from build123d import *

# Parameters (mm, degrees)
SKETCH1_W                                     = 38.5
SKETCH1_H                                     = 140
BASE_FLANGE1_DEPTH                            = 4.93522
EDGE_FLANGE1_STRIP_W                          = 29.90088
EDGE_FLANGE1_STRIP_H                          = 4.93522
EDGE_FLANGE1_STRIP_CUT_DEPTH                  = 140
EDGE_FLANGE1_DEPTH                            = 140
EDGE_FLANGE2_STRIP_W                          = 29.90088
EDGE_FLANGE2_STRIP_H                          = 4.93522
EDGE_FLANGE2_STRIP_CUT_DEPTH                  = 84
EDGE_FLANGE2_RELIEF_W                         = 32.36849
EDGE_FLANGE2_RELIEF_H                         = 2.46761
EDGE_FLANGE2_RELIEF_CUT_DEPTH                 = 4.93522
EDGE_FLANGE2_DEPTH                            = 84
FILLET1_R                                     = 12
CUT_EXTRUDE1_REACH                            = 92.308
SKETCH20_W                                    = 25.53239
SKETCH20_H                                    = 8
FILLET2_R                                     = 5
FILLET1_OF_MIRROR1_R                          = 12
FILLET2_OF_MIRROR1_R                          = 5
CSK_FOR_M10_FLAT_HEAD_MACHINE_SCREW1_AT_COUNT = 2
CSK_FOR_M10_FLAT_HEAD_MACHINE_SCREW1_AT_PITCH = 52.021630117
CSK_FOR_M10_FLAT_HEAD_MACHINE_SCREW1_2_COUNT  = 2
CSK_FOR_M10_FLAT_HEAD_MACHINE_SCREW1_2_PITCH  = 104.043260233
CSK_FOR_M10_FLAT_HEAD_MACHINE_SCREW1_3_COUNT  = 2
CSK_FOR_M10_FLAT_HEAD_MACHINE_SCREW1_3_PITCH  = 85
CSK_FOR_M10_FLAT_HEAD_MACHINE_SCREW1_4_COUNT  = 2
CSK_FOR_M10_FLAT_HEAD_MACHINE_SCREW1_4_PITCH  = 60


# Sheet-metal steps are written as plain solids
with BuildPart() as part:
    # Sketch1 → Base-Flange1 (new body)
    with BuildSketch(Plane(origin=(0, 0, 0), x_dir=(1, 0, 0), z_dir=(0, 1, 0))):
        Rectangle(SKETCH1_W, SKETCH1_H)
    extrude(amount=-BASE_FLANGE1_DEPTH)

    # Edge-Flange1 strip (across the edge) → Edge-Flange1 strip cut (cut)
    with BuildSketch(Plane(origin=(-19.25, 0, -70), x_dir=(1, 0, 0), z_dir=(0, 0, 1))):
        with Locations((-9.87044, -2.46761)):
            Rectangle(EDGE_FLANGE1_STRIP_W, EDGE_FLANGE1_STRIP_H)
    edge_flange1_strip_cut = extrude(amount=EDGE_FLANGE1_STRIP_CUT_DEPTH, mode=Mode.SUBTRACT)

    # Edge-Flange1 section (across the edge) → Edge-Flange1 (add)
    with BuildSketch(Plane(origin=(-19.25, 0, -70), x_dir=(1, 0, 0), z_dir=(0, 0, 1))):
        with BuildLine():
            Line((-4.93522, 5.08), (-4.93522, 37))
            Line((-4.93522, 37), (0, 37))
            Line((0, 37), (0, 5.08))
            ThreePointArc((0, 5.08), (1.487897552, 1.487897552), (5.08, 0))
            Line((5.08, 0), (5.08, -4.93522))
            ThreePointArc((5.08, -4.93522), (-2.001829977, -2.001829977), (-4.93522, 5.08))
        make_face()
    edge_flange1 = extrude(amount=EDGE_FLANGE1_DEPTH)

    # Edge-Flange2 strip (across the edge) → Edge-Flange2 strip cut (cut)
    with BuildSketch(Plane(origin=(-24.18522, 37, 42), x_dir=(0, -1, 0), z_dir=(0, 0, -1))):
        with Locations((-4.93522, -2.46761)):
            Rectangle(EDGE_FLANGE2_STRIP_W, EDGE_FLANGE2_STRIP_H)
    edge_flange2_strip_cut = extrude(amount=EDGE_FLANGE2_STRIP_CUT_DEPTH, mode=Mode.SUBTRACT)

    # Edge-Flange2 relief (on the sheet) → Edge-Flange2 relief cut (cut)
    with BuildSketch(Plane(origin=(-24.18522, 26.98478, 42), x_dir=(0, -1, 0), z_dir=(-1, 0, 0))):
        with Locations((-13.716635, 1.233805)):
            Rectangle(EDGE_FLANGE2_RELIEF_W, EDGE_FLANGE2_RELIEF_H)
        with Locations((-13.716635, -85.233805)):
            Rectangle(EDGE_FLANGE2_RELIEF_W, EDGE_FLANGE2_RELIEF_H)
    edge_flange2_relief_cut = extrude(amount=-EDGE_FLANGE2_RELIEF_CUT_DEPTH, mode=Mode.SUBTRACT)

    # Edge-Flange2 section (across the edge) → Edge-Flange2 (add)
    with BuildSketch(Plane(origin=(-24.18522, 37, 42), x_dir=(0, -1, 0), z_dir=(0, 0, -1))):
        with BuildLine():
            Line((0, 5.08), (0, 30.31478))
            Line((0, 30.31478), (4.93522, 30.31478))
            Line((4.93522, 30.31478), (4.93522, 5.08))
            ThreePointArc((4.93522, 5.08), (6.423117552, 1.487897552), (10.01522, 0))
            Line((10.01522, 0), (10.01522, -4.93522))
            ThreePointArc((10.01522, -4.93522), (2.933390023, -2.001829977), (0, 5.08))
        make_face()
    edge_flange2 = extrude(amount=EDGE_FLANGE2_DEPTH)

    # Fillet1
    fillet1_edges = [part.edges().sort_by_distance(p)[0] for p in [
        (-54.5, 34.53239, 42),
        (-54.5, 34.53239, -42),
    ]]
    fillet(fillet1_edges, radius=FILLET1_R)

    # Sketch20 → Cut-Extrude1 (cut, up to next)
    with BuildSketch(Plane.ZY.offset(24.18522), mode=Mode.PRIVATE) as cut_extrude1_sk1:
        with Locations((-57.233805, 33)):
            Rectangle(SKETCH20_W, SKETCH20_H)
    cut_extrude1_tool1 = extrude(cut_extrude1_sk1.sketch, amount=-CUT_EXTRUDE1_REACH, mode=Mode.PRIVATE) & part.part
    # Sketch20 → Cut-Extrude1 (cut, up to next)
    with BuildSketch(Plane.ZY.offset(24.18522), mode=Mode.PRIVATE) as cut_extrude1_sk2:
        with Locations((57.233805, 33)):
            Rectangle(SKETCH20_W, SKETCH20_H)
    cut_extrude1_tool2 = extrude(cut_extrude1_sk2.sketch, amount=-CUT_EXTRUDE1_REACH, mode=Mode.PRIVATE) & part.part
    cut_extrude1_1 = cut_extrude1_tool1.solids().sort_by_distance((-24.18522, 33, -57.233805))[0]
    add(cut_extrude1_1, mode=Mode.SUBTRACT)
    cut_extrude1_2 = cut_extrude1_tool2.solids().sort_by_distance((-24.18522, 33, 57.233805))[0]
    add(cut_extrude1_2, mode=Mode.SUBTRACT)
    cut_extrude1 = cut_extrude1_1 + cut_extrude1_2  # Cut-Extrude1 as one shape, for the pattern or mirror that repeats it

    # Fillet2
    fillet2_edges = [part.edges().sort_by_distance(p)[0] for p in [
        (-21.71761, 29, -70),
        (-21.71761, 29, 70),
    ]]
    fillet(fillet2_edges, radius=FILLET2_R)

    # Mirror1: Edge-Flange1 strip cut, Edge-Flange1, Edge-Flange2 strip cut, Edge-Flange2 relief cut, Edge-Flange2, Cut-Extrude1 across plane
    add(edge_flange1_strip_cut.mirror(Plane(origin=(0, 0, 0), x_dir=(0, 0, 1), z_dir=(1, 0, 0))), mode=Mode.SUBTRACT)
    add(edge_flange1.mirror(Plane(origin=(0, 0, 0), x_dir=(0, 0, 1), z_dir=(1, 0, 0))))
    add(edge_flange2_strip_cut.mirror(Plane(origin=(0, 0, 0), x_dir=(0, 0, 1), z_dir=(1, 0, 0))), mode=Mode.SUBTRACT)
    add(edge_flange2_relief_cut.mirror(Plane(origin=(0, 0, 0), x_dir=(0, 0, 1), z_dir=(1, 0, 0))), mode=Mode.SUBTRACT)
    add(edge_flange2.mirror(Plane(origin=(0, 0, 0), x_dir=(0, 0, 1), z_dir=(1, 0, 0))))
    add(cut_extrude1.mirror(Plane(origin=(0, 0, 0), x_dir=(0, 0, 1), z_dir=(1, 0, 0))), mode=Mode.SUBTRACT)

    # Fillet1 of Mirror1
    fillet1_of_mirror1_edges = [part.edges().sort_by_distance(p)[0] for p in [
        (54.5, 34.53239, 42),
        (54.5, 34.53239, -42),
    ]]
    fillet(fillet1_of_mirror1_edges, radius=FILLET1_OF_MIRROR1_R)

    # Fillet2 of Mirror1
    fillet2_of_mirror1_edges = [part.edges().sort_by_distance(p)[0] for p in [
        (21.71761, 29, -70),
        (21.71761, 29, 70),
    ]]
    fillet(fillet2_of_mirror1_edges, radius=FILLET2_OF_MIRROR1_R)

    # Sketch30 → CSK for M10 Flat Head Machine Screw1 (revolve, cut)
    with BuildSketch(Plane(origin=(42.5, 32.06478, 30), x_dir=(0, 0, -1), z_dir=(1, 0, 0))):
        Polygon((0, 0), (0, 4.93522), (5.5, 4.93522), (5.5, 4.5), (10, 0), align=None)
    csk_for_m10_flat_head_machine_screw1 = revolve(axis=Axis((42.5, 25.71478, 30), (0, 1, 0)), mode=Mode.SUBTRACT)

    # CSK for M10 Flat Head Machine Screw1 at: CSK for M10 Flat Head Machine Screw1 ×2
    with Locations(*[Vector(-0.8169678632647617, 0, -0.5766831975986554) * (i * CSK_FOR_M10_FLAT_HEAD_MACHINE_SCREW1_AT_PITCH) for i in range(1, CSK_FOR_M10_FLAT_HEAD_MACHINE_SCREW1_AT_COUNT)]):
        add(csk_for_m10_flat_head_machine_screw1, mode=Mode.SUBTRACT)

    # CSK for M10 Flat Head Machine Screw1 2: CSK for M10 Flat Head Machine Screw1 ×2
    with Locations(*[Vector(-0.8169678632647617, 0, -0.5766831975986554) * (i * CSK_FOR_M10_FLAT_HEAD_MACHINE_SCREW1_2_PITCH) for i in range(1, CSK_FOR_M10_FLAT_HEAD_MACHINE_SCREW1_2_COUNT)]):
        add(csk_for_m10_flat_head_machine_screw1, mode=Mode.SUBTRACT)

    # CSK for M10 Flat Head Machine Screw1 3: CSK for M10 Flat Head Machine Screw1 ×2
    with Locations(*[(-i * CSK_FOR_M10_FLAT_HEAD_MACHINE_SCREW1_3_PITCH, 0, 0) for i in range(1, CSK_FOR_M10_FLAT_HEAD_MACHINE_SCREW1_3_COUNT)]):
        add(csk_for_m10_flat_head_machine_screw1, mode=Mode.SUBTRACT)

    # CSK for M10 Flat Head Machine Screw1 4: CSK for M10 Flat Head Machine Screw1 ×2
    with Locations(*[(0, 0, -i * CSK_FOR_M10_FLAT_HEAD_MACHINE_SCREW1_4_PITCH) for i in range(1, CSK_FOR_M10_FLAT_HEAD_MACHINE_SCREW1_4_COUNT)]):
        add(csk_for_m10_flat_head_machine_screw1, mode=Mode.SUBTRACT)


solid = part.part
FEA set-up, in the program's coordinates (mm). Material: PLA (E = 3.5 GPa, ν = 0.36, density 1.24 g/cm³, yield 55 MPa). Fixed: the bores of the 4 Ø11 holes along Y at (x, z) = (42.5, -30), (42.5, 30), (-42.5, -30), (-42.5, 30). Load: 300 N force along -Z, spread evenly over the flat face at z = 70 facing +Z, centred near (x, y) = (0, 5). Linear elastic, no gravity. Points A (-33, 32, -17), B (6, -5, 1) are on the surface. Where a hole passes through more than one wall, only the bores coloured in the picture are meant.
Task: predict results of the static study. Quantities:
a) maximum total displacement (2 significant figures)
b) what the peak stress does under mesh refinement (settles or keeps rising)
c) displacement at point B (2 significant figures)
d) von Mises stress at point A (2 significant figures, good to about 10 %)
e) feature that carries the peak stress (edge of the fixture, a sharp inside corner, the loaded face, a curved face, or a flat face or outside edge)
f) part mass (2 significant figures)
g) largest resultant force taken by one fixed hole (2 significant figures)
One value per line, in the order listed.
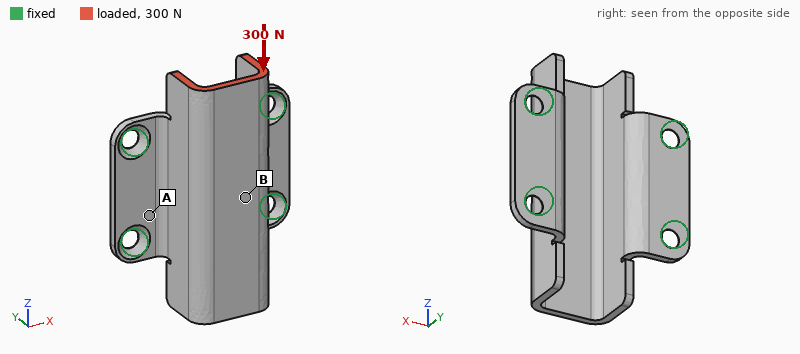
0.29 mm
keeps rising
0.14 mm
3.3 MPa
edge of the fixture
120 g
130 N
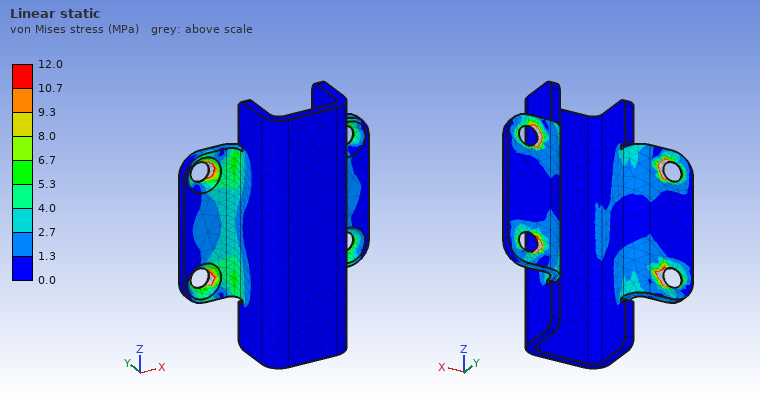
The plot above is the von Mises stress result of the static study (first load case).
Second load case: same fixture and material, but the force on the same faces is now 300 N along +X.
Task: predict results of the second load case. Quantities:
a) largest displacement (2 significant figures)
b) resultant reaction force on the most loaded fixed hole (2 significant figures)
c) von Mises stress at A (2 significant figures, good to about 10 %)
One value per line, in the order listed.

1.3 mm
140 N
3.9 MPa
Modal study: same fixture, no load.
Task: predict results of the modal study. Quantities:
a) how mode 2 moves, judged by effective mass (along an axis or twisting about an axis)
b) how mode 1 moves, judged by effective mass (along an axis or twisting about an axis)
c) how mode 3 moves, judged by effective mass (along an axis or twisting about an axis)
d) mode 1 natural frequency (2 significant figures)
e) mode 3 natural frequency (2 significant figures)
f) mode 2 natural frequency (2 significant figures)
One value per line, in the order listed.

twisting about Y
along Z
along X
540 Hz
670 Hz
610 Hz
